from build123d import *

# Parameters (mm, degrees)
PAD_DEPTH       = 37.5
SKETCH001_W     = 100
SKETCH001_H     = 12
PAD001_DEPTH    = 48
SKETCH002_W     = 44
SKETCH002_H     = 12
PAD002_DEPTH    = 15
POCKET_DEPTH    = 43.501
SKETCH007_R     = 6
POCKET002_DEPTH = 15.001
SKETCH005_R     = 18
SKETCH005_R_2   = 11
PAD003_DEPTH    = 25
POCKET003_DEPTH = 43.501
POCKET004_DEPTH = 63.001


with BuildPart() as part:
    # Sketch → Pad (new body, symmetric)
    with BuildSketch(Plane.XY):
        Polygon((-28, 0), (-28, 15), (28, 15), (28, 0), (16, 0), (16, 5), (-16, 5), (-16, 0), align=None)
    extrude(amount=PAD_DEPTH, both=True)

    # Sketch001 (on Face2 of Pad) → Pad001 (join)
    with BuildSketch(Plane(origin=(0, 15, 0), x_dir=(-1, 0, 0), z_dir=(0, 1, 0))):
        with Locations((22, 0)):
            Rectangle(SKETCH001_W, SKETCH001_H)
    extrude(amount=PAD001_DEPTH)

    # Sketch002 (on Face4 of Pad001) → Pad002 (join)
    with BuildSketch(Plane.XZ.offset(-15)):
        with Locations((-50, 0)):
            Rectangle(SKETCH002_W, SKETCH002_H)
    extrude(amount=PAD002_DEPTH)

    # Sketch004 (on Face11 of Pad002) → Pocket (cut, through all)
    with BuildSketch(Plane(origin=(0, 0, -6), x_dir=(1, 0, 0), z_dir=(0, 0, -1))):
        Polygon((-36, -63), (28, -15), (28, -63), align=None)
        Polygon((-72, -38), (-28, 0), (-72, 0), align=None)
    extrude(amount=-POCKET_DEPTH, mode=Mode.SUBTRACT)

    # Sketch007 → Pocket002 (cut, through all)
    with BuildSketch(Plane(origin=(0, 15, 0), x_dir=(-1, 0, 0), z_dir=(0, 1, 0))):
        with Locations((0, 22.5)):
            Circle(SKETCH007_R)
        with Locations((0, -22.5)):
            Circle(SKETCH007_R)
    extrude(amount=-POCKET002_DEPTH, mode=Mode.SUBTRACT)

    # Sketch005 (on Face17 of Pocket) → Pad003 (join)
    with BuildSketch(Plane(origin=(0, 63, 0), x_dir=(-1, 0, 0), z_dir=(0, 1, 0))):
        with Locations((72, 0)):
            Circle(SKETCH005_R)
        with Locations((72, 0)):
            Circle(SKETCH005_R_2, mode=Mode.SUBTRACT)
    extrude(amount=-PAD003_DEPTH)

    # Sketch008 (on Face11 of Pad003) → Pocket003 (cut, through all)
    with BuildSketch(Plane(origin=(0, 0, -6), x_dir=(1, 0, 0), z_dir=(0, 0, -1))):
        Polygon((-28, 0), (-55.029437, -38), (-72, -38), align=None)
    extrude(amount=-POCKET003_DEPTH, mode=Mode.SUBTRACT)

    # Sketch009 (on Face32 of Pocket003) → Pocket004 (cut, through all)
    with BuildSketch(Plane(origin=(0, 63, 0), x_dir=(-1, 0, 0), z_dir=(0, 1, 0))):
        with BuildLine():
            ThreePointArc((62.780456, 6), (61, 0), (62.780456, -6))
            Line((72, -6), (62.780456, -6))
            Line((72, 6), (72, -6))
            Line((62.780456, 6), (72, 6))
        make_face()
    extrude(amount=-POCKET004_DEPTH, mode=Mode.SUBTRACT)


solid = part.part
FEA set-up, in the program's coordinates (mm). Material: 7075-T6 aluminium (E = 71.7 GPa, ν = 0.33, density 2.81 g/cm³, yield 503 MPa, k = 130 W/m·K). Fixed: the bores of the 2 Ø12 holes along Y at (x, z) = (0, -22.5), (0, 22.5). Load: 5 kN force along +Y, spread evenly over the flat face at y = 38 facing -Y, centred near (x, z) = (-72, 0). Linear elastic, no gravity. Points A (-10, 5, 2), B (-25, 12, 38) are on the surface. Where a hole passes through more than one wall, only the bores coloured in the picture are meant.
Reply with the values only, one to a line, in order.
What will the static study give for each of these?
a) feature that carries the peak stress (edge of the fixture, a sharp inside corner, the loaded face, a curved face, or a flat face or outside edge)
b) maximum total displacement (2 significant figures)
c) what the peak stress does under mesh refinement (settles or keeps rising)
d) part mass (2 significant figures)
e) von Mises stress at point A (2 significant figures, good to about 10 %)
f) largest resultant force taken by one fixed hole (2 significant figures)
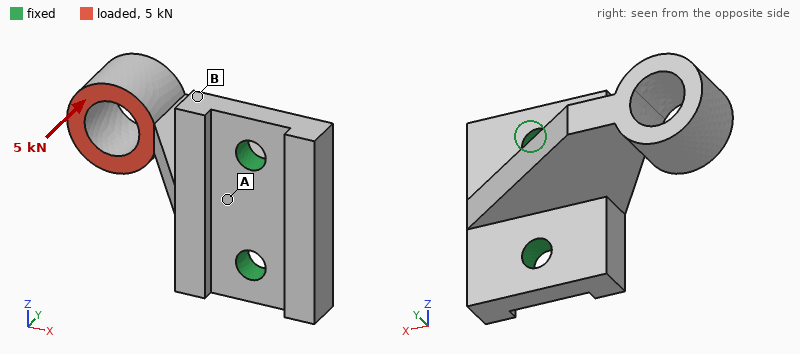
edge of the fixture
0.78 mm
keeps rising
260 g
77 MPa
3.3 kN
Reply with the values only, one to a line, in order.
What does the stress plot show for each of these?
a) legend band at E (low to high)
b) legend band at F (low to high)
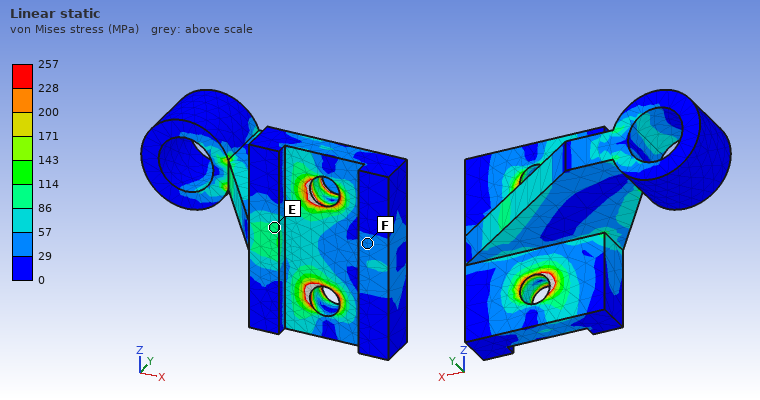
86 to 114 MPa
29 to 57 MPa
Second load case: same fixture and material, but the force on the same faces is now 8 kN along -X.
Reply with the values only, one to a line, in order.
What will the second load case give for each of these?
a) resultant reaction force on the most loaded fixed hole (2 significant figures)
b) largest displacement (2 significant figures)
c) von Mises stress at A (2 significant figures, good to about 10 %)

4.0 kN
0.29 mm
34 MPa
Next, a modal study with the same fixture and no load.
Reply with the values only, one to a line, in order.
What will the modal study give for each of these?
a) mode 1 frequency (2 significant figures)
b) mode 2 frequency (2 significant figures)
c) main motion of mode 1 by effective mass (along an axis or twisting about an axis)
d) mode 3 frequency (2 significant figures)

1200 Hz
1800 Hz
along Z
3600 Hz
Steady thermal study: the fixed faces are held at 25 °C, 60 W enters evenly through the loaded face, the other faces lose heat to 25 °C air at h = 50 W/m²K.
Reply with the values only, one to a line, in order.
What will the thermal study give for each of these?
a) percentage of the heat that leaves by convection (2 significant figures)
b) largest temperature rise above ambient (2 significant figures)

39 %
74 K
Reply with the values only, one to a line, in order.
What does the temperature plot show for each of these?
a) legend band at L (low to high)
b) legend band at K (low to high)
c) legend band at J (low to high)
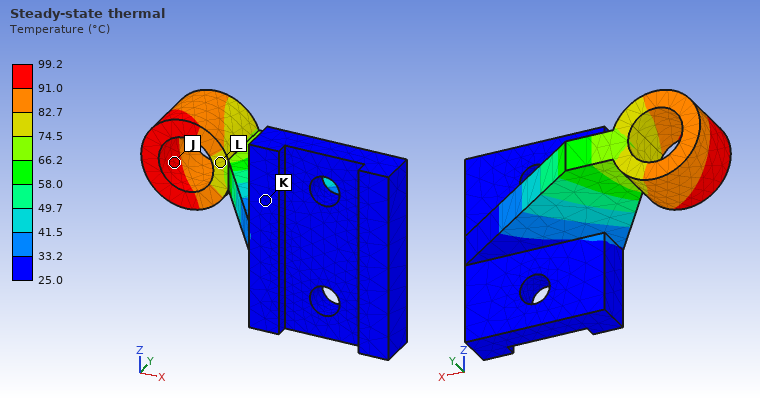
74.5 to 82.7 °C
25.0 to 33.2 °C
91.0 to 99.2 °C
